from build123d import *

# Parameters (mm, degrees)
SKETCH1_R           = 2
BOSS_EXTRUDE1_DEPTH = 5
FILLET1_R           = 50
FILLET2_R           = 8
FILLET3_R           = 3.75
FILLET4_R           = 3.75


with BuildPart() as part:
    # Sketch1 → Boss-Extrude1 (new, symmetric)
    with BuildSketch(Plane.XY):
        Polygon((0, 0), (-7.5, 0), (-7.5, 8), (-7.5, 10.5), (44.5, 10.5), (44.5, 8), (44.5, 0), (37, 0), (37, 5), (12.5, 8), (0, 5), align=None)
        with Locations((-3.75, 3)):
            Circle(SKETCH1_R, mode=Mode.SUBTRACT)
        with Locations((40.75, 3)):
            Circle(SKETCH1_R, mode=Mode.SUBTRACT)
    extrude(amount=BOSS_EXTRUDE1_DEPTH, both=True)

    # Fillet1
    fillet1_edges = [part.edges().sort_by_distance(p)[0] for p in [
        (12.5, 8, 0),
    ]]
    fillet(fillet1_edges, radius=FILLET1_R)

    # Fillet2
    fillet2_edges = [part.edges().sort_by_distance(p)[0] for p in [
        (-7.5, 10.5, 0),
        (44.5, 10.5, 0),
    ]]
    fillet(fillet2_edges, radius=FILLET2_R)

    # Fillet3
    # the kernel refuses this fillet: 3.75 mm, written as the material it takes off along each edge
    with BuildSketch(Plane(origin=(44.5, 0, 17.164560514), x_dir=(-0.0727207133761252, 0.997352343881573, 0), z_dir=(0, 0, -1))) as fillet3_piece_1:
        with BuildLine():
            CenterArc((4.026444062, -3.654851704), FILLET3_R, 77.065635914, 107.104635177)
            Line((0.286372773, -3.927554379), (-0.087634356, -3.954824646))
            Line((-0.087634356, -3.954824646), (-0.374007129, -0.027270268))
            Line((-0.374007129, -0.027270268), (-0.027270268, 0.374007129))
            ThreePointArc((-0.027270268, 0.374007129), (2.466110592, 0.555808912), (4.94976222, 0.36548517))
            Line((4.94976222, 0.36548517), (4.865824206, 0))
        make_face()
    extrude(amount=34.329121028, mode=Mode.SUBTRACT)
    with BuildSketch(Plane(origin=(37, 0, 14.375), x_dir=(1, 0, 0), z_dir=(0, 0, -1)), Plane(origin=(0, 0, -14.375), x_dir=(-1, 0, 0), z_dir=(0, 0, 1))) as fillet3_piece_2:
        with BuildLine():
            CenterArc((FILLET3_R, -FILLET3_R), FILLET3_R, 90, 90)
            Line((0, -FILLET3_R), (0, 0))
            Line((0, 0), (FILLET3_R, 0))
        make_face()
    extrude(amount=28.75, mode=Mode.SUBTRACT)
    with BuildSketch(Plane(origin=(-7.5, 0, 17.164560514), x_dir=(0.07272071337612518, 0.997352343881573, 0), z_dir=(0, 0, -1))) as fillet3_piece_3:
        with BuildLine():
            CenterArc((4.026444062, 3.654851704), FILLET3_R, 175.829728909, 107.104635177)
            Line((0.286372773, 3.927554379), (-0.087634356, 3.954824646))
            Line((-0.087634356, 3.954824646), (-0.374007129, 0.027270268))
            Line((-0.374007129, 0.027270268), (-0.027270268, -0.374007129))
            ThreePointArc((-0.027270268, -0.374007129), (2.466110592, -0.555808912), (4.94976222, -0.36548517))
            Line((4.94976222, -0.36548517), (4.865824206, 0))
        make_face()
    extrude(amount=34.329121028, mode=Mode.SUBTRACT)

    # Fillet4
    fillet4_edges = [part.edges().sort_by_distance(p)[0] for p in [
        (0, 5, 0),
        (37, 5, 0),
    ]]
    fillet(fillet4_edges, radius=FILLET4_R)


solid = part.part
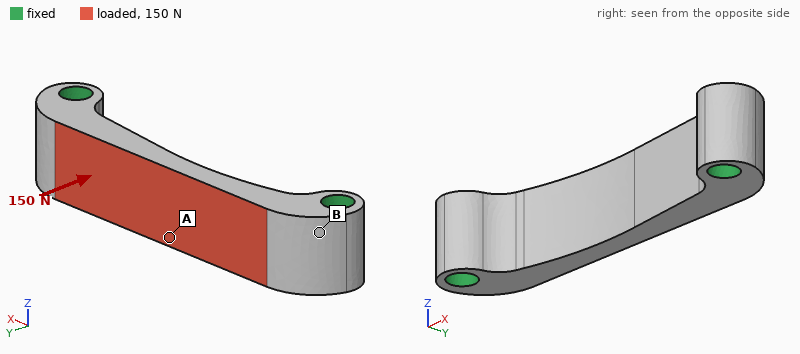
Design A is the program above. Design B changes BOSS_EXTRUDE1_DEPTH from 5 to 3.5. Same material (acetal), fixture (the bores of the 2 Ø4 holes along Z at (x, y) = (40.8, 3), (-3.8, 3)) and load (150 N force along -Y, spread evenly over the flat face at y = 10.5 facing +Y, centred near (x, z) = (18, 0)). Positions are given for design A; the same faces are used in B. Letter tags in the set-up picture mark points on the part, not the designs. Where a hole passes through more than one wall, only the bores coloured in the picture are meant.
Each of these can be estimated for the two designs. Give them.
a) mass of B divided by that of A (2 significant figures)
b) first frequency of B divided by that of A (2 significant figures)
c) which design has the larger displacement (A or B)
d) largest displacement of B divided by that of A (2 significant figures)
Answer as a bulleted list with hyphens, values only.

- 0.70
- 0.99
- B
- 1.4
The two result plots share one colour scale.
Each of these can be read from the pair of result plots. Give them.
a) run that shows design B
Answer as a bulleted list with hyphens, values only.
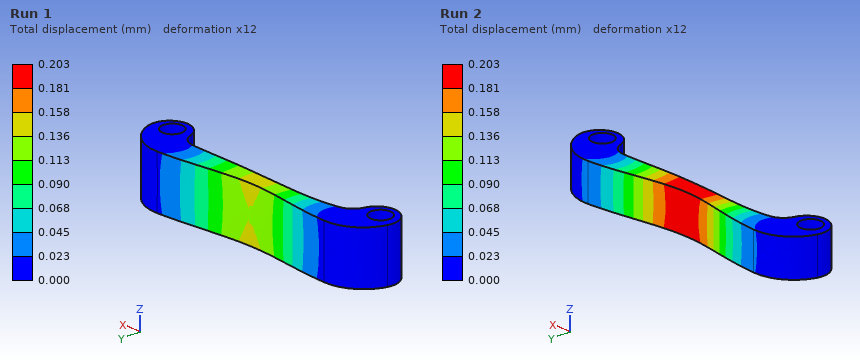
- Run 2
